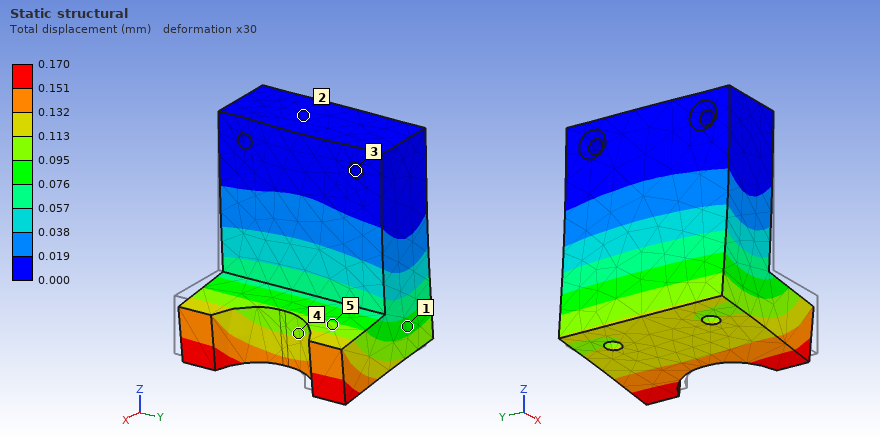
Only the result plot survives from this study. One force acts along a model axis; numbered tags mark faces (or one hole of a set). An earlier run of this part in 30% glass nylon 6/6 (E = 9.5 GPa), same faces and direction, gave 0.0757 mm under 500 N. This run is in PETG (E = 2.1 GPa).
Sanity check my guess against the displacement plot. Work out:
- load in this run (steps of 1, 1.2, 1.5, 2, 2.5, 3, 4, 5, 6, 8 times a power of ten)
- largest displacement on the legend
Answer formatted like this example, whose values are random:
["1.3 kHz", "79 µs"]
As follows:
["250 N", "0.170 mm"]
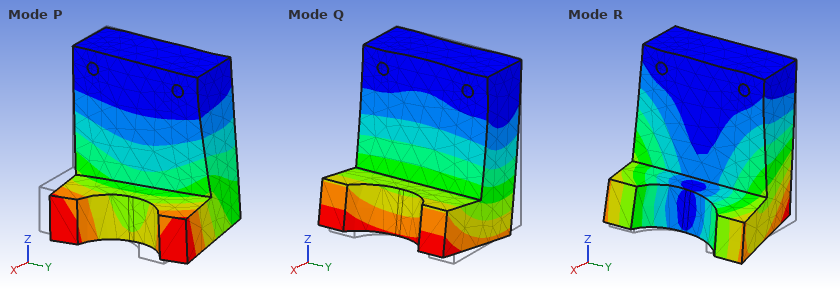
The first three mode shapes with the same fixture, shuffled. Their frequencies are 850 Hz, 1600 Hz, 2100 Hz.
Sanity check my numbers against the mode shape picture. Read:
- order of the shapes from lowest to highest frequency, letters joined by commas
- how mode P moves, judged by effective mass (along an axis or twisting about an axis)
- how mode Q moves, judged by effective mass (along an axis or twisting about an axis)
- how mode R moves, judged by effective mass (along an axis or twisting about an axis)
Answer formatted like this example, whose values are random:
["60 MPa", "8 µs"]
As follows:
["Q, P, R", "along Y", "along X", "along Y"]
